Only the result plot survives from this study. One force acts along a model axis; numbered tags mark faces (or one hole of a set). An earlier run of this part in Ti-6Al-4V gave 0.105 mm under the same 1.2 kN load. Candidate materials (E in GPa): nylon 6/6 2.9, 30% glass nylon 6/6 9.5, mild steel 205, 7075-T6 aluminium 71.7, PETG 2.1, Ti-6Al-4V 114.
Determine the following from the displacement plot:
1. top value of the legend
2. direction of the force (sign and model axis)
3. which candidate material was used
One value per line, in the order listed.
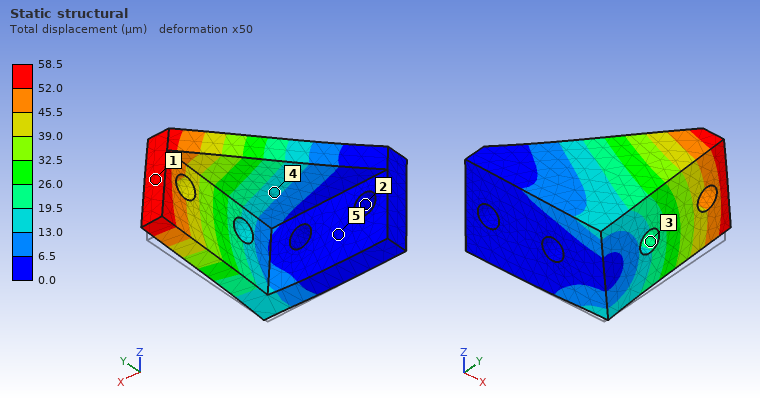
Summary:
58.5 µm
+Z
mild steel
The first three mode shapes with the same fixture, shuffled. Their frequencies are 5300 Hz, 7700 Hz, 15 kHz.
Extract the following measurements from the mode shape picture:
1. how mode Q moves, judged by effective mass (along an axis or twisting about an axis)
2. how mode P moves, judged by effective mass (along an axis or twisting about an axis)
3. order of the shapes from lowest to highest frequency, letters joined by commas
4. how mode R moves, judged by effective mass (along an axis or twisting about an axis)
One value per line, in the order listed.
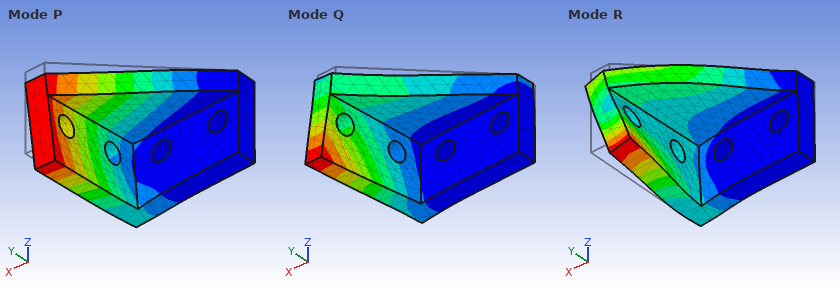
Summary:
along X
along Z
P, Q, R
along Y
